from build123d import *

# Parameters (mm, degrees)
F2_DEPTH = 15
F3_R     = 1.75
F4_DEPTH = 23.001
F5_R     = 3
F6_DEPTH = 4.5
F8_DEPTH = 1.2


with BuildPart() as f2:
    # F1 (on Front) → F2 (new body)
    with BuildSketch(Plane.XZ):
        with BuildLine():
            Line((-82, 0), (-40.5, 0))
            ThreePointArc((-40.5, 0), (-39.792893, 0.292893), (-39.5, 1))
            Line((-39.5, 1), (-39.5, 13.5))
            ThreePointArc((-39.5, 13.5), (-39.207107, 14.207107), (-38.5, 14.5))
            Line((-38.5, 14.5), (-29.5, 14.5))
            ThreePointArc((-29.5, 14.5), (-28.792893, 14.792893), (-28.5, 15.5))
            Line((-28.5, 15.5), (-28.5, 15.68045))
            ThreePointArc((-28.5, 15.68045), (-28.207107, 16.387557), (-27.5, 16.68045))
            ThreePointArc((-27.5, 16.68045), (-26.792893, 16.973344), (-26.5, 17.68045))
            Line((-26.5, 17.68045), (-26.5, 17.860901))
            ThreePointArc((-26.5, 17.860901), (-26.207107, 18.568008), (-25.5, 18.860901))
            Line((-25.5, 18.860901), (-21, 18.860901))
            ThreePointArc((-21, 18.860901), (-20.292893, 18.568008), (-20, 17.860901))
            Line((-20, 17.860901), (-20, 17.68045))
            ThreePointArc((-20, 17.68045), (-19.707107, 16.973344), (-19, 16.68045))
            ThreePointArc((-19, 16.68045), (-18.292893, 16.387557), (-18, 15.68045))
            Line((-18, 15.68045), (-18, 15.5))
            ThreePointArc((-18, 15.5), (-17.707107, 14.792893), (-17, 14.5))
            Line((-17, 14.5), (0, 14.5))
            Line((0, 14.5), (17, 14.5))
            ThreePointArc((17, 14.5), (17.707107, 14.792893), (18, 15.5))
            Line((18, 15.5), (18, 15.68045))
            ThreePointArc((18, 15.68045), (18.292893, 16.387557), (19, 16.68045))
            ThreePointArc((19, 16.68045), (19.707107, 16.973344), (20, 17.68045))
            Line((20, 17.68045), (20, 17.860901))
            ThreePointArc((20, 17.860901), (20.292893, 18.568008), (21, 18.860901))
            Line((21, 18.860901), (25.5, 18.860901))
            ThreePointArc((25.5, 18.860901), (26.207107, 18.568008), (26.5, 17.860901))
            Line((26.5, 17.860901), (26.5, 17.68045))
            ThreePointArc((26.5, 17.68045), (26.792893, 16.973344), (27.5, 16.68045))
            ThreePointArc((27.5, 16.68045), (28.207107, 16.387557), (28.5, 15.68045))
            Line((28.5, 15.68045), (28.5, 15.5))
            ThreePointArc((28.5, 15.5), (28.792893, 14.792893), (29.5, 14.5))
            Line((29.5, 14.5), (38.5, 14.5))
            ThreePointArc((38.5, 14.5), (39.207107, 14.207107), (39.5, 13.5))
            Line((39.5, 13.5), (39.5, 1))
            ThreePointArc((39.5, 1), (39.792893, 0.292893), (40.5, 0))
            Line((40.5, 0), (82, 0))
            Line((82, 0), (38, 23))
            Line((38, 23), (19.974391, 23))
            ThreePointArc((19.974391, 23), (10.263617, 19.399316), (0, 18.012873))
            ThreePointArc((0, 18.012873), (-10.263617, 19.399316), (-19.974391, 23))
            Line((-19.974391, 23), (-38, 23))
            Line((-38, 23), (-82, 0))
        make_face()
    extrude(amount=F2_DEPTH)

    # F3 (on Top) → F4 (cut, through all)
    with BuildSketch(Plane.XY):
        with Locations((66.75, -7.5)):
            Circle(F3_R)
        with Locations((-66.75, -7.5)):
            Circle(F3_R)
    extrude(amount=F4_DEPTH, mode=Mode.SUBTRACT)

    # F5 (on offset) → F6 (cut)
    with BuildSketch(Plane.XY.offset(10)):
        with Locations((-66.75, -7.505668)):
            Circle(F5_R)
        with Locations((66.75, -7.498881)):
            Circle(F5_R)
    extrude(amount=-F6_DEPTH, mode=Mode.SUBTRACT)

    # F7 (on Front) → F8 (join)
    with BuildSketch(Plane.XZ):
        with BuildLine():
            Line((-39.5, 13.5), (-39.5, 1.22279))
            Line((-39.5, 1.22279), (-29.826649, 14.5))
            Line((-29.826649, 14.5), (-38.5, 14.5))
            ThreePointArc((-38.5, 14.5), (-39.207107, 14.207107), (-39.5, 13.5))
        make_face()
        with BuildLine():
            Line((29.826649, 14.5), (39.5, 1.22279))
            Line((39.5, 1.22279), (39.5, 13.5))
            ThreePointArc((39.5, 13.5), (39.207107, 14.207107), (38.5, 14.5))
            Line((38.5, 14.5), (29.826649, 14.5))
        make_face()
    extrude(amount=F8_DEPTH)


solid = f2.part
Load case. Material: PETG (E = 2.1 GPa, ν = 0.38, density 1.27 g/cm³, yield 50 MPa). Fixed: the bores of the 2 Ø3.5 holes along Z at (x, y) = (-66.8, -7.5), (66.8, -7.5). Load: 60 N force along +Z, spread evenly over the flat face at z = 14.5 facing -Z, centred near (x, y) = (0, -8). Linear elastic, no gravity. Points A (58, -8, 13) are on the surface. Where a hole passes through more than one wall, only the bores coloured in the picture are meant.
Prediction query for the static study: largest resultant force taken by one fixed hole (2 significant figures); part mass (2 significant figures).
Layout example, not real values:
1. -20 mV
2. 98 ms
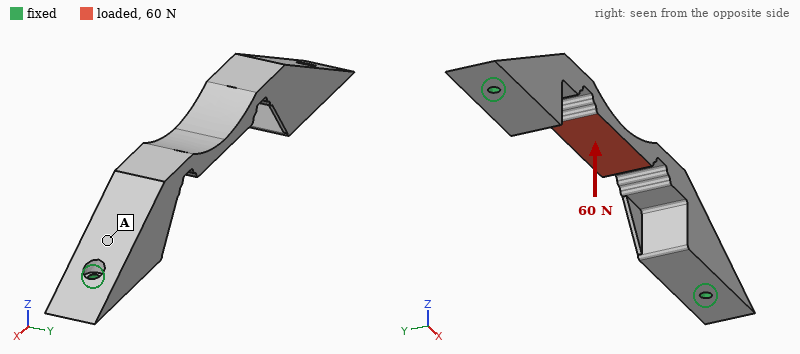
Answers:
1. 59 N
2. 27 g
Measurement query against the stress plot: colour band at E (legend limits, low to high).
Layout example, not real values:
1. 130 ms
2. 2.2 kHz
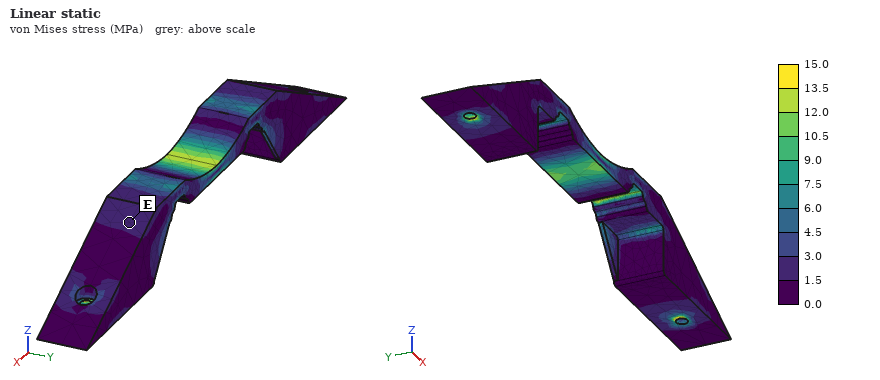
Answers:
1. 1.5 to 3.0 MPa
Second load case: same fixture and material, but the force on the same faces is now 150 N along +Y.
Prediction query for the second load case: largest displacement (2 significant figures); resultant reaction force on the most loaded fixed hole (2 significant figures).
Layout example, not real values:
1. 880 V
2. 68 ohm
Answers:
1. 1.3 mm
2. 75 N
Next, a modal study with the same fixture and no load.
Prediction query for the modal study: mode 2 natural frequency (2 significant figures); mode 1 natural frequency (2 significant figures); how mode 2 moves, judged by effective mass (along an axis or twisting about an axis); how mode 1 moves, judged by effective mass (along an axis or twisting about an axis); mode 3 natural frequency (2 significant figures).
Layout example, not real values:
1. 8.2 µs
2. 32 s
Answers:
1. 690 Hz
2. 640 Hz
3. along Z
4. along Y
5. 830 Hz
